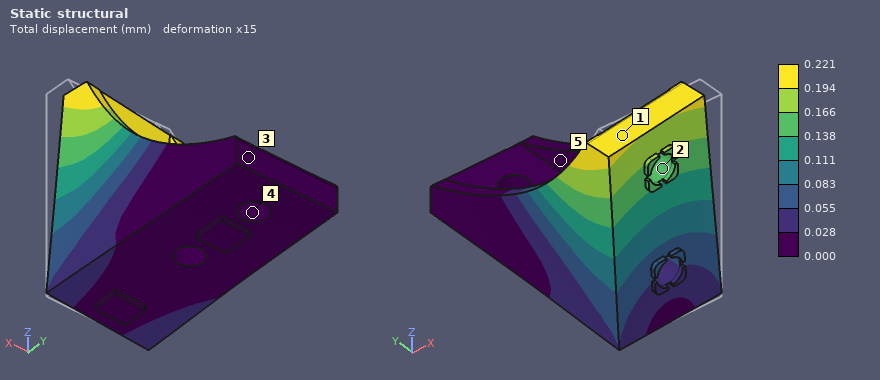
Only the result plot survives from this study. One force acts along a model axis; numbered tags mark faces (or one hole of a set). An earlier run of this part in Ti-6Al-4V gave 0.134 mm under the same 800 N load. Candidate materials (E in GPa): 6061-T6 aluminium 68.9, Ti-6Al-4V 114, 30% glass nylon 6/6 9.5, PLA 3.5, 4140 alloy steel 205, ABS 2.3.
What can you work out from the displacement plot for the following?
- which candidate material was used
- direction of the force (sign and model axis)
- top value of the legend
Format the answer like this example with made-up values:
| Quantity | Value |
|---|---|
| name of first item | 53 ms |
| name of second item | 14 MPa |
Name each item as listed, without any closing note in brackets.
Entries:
| Quantity | Value |
|---|---|
| which candidate material was used | 6061-T6 aluminium |
| direction of the force | -X |
| top value of the legend | 0.221 mm |
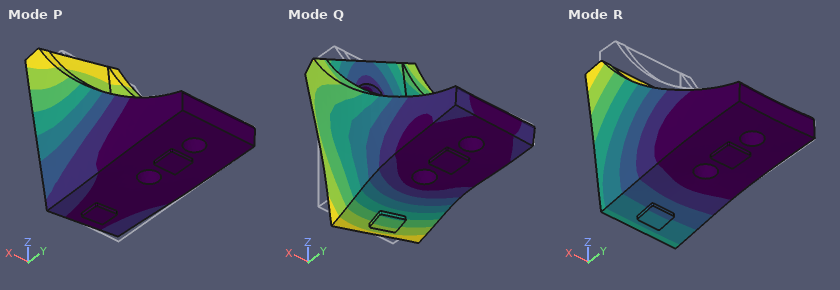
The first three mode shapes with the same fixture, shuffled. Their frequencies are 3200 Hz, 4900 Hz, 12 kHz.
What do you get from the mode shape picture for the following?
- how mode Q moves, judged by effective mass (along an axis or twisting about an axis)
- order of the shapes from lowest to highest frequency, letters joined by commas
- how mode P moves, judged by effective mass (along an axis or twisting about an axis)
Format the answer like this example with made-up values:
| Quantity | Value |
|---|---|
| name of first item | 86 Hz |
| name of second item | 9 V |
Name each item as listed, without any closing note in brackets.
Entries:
| Quantity | Value |
|---|---|
| how mode Q moves, judged by effective mass | along X |
| order of the shapes from lowest to highest frequency, letters joined by commas | P, R, Q |
| how mode P moves, judged by effective mass | along X |
